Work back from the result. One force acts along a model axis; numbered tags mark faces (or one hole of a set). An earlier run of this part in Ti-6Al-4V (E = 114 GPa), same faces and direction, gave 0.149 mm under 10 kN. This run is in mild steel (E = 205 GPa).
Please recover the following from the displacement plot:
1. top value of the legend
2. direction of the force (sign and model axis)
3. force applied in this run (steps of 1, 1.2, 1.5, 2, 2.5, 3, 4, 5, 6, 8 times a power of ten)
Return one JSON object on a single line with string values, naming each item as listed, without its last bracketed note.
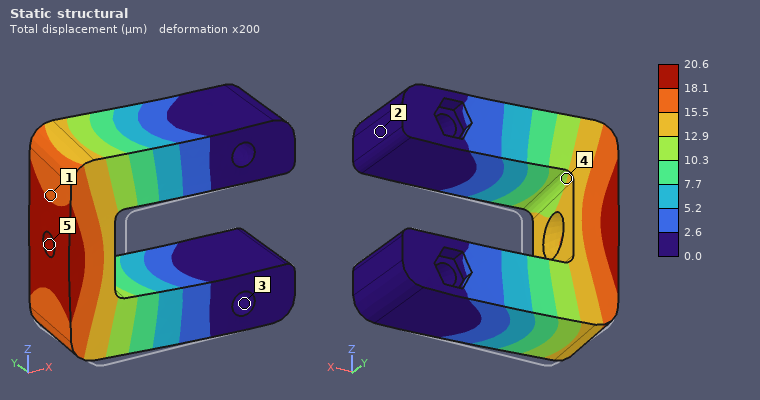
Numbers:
{"top value of the legend": "20.6 µm", "direction of the force": "+Y", "force applied in this run": "2.5 kN"}
